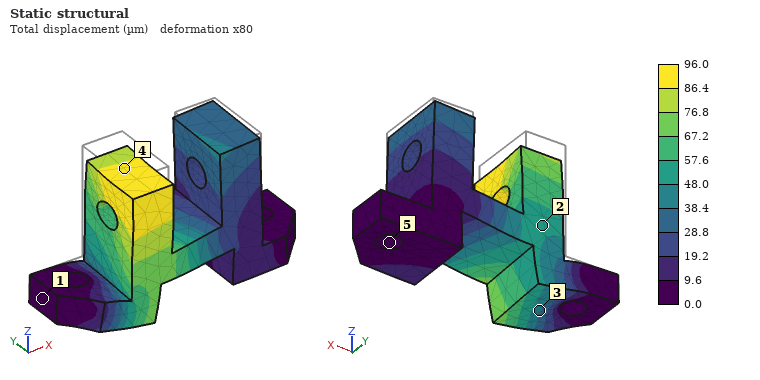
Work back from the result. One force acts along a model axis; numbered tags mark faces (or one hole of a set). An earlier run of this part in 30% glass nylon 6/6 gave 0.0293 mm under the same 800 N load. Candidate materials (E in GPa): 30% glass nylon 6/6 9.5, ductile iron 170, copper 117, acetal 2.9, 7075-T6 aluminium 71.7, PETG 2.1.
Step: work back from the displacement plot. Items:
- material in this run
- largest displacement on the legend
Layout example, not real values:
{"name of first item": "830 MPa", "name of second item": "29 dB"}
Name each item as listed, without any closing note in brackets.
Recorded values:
{"material in this run": "acetal", "largest displacement on the legend": "96.0 µm"}
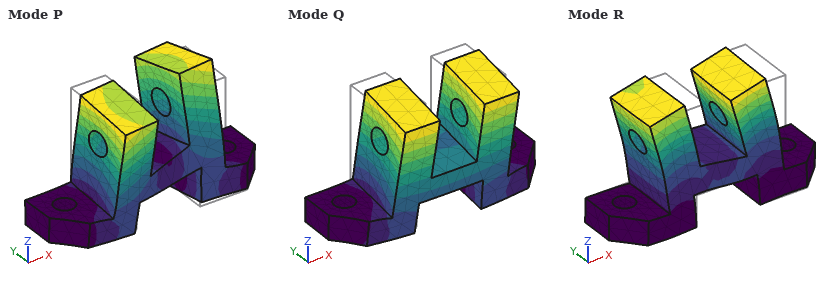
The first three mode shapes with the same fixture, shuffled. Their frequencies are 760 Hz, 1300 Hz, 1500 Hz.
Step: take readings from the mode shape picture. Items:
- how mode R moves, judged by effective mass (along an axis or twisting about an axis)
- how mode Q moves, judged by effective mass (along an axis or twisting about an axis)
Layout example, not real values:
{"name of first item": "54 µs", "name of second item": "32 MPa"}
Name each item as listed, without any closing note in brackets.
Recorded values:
{"how mode R moves, judged by effective mass": "along X", "how mode Q moves, judged by effective mass": "along Y"}
